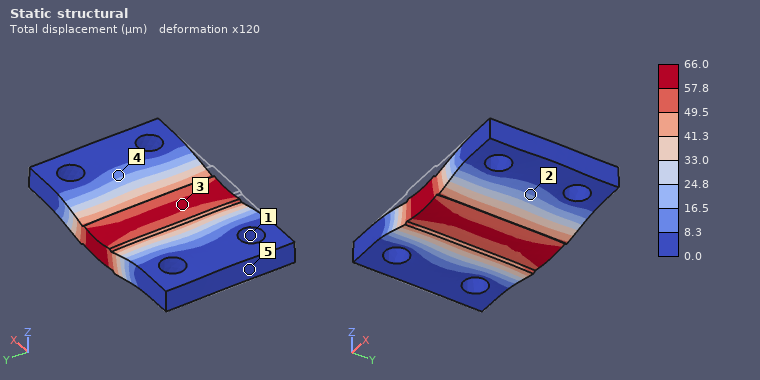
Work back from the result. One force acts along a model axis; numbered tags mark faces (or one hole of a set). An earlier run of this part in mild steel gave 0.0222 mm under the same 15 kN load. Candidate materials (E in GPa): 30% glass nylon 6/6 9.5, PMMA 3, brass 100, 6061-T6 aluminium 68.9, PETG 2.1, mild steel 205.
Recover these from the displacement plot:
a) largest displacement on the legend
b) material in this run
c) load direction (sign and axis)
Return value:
66.0 µm
6061-T6 aluminium
-Z
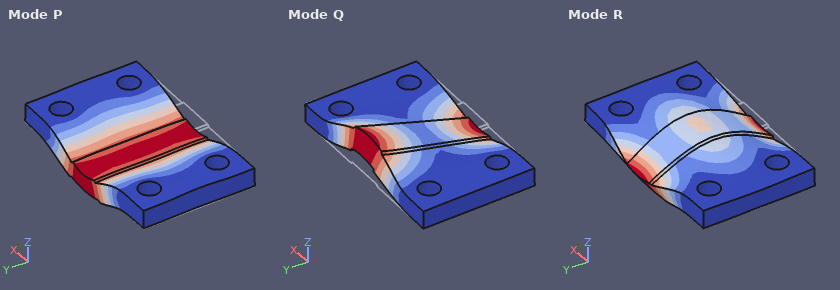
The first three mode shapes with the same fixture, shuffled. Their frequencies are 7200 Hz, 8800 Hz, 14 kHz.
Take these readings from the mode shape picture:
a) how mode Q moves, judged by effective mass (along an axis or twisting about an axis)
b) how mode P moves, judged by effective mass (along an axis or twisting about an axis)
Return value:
twisting about X
along Z
